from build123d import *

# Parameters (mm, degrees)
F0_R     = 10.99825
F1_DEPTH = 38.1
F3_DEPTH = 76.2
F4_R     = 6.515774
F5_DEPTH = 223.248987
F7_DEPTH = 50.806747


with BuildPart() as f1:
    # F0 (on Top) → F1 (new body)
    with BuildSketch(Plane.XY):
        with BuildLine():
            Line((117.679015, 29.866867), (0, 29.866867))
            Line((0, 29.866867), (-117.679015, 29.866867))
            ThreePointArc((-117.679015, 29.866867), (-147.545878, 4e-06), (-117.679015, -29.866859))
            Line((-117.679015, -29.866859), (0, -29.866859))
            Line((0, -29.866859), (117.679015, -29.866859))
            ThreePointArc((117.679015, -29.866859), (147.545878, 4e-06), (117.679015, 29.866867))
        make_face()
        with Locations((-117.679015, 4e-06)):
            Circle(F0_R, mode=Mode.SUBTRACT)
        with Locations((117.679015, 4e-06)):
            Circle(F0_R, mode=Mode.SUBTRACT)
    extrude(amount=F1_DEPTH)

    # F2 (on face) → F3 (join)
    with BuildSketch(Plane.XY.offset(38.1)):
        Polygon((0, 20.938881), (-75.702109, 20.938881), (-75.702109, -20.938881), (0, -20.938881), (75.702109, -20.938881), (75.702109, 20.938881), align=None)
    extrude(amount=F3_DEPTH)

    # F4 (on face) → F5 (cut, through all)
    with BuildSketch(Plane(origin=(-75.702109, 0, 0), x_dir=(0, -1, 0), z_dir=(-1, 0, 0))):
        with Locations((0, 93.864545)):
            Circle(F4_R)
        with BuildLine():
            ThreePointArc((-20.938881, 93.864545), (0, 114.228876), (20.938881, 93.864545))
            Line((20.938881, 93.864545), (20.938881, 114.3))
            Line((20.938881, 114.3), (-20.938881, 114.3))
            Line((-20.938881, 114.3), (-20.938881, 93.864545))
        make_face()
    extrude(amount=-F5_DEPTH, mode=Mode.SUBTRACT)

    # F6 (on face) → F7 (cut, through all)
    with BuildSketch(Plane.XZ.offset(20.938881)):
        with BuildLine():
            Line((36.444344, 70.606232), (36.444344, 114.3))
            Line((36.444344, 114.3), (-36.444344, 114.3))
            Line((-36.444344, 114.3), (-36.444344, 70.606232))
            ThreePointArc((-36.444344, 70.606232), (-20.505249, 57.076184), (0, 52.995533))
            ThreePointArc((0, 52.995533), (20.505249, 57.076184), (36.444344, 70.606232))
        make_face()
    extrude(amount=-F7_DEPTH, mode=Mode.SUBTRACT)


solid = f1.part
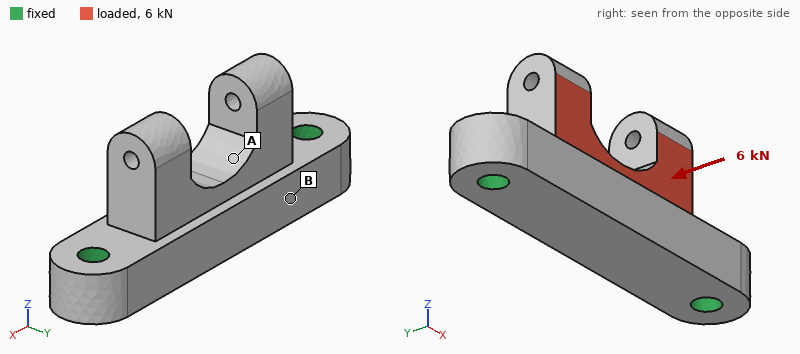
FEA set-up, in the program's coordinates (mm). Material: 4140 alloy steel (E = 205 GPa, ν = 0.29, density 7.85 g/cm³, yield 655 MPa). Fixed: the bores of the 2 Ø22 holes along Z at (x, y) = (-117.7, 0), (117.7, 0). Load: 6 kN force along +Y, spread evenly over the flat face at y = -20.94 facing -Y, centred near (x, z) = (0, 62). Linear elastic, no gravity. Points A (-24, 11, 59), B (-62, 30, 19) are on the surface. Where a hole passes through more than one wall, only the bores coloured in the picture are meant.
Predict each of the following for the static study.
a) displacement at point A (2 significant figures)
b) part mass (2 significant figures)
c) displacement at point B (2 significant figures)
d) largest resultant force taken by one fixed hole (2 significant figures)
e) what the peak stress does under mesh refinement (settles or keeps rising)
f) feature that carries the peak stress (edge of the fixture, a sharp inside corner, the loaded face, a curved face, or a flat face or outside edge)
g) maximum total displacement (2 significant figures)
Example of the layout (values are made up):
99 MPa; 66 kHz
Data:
8.6 µm; 7.1 kg; 4.0 µm; 3.0 kN; keeps rising; edge of the fixture; 16 µm
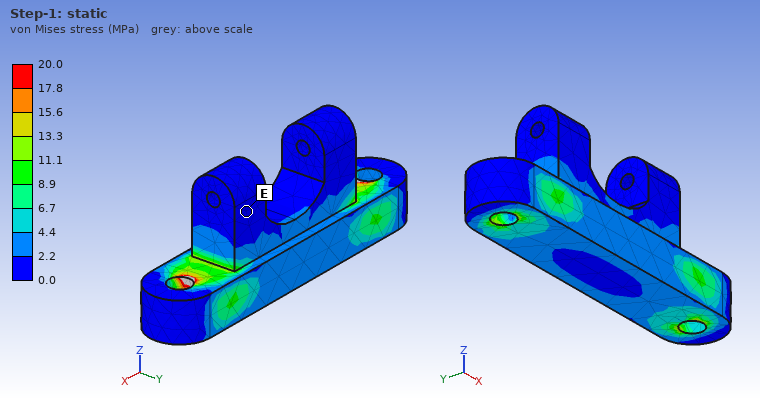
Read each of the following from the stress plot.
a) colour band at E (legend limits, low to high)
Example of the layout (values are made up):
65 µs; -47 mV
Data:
0.0 to 2.2 MPa
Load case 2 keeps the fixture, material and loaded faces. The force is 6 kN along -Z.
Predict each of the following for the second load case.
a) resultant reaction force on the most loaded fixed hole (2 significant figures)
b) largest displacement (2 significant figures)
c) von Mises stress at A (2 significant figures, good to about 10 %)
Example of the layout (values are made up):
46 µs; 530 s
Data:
3.2 kN; 8.4 µm; 2.9 MPa
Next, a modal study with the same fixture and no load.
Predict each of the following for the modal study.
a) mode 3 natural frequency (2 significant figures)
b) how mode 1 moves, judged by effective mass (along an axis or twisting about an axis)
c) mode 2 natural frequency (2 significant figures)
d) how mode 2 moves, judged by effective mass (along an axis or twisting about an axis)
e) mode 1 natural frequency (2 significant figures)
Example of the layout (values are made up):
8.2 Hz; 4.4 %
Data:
3800 Hz; along Y; 3000 Hz; along Z; 2200 Hz
